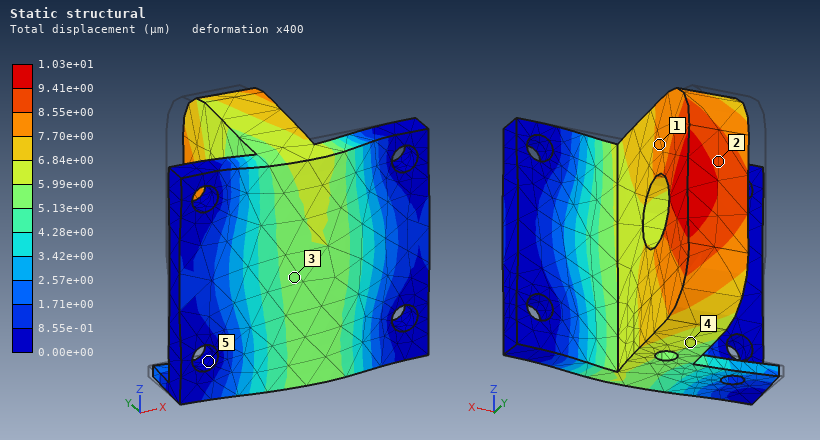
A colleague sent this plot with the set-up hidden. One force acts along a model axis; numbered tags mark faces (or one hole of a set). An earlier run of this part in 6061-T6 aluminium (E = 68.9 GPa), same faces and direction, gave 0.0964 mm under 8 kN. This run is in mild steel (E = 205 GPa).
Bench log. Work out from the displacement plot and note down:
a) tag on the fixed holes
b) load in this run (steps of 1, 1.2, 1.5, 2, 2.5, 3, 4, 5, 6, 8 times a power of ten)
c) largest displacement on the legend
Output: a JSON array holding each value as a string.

["5", "2.5 kN", "1.03e+01 µm"]
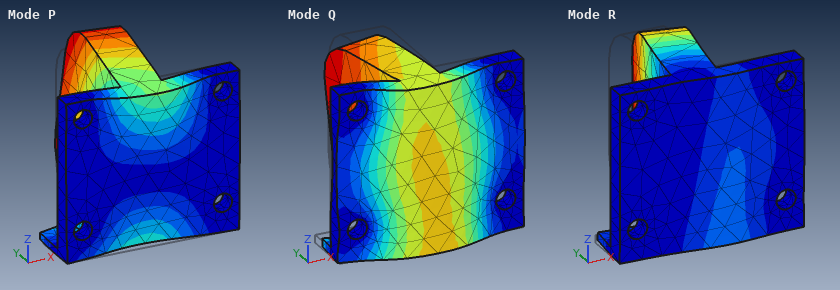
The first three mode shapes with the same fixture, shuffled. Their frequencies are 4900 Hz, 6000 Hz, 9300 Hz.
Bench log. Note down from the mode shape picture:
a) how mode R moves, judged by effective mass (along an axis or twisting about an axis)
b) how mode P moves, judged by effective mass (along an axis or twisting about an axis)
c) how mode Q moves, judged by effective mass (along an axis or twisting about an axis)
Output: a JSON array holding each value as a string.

["along X", "along Z", "along Y"]
